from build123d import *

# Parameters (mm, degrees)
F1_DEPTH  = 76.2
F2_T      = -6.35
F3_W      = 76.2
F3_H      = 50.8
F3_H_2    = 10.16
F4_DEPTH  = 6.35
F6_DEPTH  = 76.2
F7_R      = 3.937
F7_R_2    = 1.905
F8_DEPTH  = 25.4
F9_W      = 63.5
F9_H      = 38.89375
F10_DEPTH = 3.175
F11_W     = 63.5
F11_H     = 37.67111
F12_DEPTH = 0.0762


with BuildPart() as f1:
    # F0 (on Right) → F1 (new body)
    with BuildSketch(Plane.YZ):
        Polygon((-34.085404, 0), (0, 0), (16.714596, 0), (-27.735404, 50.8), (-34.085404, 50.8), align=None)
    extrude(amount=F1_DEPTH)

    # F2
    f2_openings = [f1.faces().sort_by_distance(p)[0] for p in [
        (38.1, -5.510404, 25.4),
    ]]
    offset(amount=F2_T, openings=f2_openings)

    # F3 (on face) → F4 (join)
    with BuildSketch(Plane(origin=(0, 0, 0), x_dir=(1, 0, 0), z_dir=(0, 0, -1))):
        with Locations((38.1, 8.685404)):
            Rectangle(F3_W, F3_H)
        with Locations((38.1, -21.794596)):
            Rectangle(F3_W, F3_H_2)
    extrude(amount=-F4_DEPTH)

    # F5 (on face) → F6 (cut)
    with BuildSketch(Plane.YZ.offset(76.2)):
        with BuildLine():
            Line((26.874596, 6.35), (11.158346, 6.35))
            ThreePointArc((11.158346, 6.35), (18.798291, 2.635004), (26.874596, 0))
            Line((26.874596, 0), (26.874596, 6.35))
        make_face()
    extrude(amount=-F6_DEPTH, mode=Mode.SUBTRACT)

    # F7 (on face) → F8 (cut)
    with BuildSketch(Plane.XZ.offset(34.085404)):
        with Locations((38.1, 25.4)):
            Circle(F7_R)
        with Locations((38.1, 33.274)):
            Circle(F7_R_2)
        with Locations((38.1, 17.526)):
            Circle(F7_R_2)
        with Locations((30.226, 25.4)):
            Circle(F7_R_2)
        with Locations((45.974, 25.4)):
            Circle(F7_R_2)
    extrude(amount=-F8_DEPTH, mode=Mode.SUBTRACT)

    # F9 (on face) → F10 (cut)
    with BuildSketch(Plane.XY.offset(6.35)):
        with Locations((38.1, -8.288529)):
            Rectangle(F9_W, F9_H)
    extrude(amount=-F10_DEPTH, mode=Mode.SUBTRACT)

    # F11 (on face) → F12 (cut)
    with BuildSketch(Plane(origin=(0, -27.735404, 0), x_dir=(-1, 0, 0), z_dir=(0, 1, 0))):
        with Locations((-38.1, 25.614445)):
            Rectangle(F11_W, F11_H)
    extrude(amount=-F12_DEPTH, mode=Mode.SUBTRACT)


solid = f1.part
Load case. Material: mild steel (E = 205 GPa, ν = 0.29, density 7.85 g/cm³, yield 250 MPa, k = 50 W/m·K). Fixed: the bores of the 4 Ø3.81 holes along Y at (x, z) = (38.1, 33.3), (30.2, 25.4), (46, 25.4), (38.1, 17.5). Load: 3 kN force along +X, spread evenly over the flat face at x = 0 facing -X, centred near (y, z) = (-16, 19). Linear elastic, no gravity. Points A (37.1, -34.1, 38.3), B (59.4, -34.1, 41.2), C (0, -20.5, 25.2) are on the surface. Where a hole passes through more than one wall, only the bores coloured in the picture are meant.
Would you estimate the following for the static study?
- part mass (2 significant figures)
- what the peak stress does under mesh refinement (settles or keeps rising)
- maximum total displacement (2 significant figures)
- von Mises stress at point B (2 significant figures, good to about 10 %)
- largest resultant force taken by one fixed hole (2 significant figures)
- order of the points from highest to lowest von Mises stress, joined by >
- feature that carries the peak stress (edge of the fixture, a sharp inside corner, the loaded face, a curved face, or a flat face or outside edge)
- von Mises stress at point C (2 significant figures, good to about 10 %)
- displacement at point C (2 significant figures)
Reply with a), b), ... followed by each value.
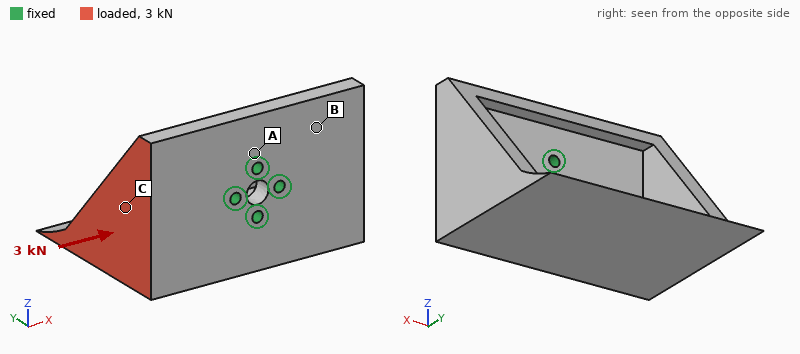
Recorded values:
a) 390 g
b) keeps rising
c) 93 µm
d) 32 MPa
e) 1.6 kN
f) B > C > A
g) edge of the fixture
h) 20 MPa
i) 41 µm
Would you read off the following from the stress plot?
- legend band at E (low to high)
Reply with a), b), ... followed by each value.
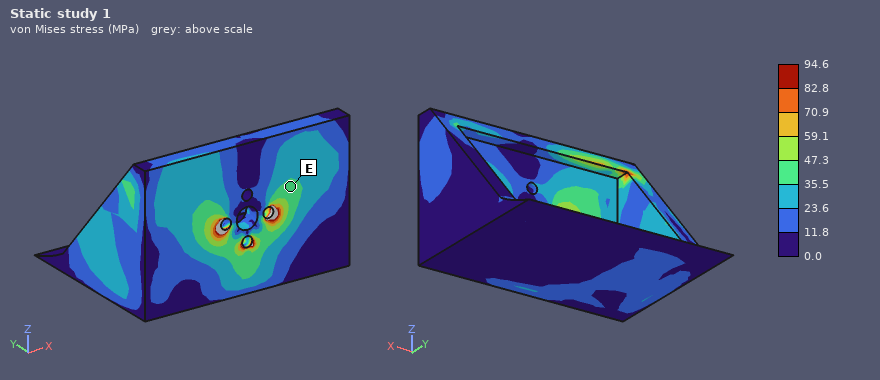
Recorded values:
a) 35.5 to 47.3 MPa
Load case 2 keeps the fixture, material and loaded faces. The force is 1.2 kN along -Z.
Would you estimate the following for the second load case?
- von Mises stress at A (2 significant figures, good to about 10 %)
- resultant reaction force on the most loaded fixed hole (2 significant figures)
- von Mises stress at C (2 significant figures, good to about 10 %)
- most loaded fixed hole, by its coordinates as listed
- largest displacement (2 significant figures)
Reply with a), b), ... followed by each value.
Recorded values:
a) 33 MPa
b) 1.7 kN
c) 11 MPa
d) (30.2, 25.4)
e) 57 µm
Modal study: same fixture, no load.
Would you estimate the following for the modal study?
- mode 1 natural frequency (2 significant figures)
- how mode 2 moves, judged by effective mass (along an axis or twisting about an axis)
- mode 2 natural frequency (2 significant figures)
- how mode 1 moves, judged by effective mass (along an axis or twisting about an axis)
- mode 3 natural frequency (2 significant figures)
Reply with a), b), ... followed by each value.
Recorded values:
a) 1700 Hz
b) along Z
c) 2100 Hz
d) along X
e) 3100 Hz
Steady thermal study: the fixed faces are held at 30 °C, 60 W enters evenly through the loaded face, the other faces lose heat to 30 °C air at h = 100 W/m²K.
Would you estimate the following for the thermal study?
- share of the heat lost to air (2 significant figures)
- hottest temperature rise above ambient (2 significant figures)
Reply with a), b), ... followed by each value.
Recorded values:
a) 61 %
b) 72 K
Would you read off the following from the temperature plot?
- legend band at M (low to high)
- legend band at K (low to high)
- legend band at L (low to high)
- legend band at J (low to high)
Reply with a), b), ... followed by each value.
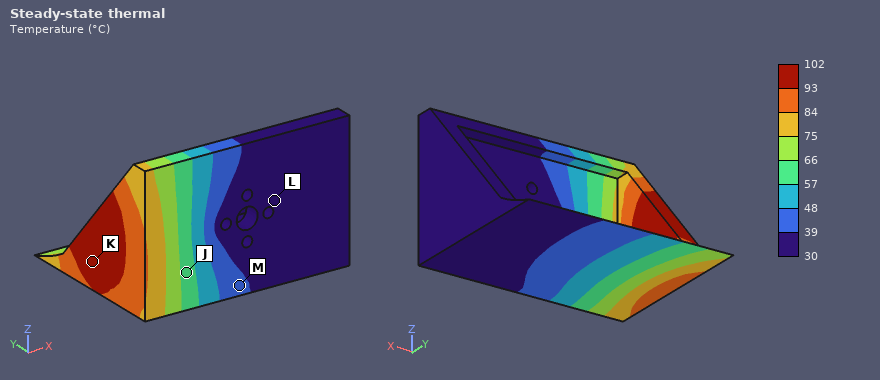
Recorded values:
a) 39 to 48 °C
b) 93 to 102 °C
c) 30 to 39 °C
d) 57 to 66 °C
